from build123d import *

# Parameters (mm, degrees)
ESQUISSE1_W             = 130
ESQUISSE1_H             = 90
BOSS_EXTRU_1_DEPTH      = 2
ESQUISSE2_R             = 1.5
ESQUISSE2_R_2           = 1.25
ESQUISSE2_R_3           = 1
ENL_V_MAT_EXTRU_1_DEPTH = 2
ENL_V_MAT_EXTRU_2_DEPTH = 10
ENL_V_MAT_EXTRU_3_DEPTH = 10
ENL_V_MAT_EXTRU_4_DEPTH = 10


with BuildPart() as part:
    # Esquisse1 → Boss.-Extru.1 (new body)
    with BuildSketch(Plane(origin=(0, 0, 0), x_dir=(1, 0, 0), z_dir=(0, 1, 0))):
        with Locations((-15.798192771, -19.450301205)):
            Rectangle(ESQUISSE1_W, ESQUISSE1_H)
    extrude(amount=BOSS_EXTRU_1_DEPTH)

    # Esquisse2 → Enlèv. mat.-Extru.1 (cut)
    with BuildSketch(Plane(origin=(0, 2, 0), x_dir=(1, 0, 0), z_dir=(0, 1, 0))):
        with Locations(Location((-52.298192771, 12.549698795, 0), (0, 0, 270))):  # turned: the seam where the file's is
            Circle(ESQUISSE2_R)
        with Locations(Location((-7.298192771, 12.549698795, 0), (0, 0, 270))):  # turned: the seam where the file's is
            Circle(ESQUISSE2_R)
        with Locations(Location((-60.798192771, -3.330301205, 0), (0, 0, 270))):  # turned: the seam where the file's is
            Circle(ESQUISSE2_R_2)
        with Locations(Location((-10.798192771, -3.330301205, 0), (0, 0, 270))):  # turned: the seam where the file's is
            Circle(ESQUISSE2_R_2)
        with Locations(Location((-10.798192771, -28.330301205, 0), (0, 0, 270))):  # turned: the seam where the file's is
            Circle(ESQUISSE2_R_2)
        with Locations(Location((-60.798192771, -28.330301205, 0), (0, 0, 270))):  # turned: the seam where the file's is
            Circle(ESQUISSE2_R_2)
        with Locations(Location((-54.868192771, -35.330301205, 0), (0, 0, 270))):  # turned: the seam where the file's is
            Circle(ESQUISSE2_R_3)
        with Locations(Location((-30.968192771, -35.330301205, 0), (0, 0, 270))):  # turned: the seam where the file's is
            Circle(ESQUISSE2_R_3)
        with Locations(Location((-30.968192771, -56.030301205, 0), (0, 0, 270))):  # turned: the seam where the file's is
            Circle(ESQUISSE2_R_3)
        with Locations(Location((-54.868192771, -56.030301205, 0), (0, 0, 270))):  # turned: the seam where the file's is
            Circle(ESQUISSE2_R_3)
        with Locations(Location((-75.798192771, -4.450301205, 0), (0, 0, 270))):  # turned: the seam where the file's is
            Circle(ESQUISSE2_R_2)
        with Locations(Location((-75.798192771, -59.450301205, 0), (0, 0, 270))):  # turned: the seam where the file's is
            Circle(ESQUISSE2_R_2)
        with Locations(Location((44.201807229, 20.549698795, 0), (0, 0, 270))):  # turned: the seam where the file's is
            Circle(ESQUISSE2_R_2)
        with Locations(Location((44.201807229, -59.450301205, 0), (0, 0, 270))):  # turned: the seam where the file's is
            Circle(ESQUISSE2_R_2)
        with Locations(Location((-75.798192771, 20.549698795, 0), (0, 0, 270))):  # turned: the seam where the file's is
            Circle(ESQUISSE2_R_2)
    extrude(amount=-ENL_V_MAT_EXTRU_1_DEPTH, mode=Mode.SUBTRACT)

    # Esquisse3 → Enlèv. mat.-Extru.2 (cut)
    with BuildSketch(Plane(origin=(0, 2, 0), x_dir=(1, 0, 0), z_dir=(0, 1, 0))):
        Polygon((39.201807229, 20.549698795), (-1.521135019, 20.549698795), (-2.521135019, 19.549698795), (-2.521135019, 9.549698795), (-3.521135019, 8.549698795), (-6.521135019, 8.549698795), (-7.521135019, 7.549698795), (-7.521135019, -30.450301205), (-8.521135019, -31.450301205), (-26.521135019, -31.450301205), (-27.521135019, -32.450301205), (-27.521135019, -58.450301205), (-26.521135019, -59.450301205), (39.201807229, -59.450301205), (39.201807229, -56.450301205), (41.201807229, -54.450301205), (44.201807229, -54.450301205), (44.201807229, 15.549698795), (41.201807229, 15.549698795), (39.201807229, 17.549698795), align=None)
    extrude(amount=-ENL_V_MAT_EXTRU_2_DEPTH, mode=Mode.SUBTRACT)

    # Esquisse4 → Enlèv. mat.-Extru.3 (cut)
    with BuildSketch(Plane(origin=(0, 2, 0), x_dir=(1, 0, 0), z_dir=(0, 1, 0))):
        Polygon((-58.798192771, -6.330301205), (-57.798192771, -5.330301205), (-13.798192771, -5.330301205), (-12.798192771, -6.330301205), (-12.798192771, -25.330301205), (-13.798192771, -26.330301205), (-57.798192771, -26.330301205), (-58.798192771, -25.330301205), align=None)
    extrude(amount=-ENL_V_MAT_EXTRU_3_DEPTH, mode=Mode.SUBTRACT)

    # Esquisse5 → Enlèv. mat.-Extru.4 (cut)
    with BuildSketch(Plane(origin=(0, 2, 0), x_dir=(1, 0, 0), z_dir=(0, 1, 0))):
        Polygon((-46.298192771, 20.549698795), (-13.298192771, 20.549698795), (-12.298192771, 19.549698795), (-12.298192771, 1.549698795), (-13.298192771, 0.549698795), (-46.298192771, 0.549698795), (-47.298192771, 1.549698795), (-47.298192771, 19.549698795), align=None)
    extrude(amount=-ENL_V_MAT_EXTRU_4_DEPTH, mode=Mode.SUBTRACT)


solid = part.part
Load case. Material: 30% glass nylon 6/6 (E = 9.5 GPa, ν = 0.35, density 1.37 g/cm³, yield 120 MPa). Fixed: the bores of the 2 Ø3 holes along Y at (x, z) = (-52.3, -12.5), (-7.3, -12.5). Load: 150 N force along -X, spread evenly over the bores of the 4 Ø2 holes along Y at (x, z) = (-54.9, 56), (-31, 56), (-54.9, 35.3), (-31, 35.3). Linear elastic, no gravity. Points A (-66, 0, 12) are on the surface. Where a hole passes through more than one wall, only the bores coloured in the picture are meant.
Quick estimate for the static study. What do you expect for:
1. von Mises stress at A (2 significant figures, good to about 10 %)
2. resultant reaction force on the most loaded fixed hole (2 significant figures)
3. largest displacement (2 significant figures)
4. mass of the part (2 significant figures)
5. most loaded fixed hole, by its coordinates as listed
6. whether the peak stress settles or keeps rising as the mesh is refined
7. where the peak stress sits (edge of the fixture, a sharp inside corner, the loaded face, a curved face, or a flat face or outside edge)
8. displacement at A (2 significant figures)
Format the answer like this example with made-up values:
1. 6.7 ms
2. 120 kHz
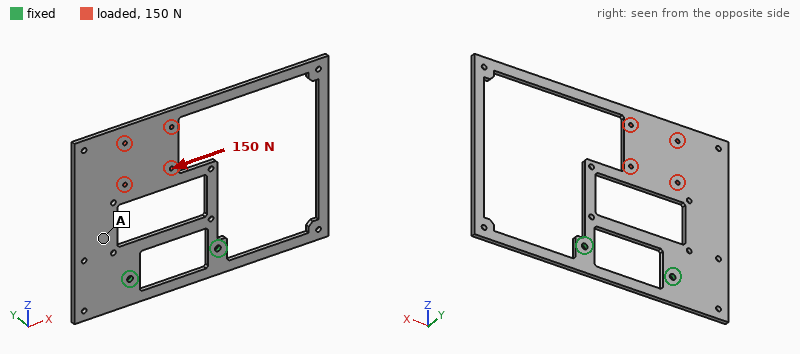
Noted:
1. 6.5 MPa
2. 210 N
3. 1.1 mm
4. 15 g
5. (-52.3, -12.5)
6. keeps rising
7. edge of the fixture
8. 0.35 mm
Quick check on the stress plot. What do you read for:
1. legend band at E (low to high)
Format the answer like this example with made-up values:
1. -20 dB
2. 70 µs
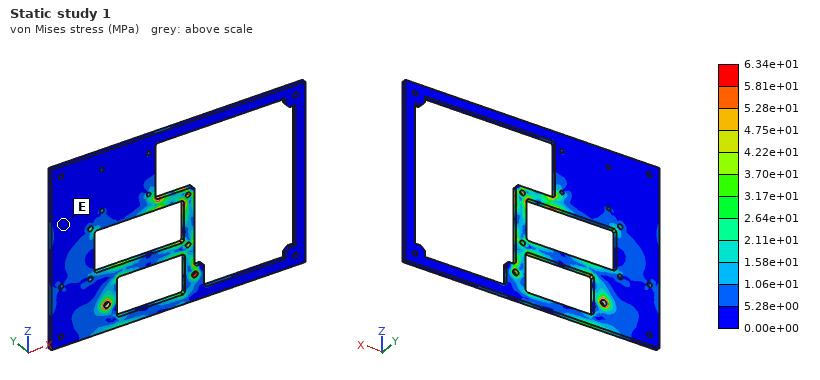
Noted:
1. 0.00e+00 to 5.28e+00 MPa
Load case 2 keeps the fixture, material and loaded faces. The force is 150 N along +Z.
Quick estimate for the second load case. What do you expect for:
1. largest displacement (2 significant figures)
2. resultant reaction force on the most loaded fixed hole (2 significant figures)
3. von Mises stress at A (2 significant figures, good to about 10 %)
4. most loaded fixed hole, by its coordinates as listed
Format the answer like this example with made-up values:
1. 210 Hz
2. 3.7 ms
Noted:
1. 0.24 mm
2. 110 N
3. 5.7 MPa
4. (-52.3, -12.5)
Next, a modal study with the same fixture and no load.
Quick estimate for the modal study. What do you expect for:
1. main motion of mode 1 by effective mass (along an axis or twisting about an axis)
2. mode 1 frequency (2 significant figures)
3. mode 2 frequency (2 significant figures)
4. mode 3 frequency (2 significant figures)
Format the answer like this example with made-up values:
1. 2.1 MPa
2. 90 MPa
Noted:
1. along Y
2. 73 Hz
3. 110 Hz
4. 210 Hz
